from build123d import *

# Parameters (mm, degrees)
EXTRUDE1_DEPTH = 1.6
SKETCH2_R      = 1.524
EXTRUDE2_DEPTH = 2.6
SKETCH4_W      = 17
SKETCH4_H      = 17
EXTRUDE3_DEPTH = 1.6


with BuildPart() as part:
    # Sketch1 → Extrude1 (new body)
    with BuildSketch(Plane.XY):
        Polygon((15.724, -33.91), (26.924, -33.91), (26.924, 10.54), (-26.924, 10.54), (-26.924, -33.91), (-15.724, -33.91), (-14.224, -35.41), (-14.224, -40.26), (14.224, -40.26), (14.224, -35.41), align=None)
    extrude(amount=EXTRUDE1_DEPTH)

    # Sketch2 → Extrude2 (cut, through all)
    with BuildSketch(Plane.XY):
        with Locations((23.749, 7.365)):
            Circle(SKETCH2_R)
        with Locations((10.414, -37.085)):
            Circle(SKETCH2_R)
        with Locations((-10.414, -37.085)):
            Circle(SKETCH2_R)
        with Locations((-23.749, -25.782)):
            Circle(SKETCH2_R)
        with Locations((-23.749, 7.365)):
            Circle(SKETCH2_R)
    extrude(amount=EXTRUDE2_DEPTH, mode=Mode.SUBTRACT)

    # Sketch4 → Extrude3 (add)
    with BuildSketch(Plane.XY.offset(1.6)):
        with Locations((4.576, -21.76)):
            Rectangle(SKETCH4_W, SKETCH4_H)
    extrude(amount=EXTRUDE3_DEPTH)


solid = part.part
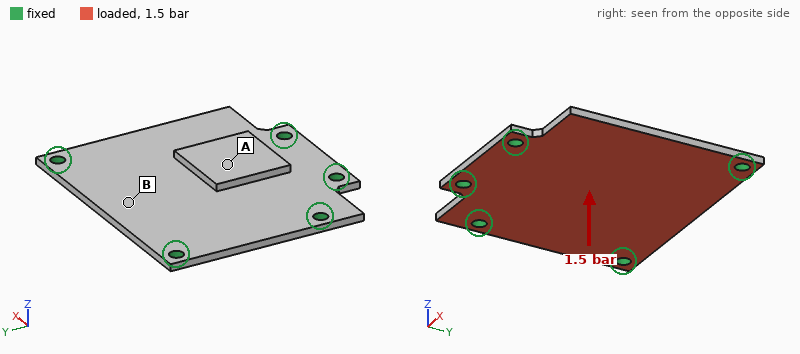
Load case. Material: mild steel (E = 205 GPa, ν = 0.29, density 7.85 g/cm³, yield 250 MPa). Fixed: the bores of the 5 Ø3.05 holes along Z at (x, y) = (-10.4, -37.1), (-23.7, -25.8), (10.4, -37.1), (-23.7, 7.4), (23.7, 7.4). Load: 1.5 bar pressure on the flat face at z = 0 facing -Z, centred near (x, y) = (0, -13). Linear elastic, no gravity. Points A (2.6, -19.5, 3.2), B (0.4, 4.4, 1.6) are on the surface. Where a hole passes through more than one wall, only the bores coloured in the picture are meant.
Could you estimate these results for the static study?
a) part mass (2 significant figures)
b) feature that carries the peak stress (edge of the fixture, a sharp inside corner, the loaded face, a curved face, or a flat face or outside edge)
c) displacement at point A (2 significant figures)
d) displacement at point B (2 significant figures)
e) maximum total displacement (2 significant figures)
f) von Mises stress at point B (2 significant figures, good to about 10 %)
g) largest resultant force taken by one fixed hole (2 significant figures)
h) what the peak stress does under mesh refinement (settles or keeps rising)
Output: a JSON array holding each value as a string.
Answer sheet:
["36 g", "edge of the fixture", "24 µm", "34 µm", "37 µm", "33 MPa", "110 N", "keeps rising"]
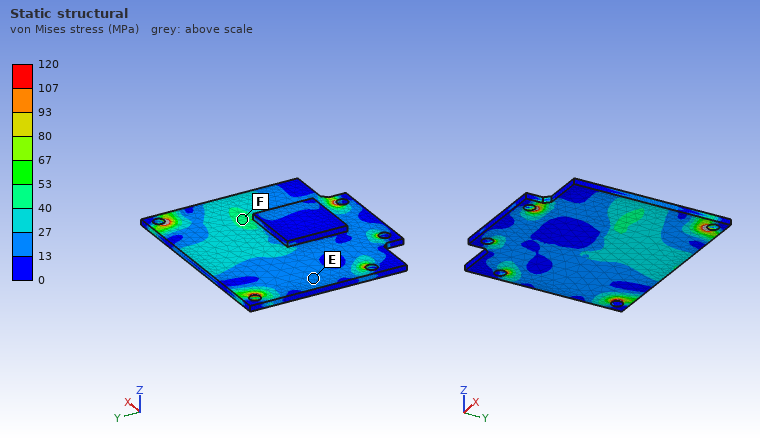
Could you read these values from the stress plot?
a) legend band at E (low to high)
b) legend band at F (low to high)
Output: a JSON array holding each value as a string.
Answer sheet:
["13 to 27 MPa", "40 to 53 MPa"]
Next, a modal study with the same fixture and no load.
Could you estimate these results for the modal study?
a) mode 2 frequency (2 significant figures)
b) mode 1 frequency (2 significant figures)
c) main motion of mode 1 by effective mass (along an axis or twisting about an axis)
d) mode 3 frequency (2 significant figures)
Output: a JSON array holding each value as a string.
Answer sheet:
["4400 Hz", "3200 Hz", "along Z", "6400 Hz"]
